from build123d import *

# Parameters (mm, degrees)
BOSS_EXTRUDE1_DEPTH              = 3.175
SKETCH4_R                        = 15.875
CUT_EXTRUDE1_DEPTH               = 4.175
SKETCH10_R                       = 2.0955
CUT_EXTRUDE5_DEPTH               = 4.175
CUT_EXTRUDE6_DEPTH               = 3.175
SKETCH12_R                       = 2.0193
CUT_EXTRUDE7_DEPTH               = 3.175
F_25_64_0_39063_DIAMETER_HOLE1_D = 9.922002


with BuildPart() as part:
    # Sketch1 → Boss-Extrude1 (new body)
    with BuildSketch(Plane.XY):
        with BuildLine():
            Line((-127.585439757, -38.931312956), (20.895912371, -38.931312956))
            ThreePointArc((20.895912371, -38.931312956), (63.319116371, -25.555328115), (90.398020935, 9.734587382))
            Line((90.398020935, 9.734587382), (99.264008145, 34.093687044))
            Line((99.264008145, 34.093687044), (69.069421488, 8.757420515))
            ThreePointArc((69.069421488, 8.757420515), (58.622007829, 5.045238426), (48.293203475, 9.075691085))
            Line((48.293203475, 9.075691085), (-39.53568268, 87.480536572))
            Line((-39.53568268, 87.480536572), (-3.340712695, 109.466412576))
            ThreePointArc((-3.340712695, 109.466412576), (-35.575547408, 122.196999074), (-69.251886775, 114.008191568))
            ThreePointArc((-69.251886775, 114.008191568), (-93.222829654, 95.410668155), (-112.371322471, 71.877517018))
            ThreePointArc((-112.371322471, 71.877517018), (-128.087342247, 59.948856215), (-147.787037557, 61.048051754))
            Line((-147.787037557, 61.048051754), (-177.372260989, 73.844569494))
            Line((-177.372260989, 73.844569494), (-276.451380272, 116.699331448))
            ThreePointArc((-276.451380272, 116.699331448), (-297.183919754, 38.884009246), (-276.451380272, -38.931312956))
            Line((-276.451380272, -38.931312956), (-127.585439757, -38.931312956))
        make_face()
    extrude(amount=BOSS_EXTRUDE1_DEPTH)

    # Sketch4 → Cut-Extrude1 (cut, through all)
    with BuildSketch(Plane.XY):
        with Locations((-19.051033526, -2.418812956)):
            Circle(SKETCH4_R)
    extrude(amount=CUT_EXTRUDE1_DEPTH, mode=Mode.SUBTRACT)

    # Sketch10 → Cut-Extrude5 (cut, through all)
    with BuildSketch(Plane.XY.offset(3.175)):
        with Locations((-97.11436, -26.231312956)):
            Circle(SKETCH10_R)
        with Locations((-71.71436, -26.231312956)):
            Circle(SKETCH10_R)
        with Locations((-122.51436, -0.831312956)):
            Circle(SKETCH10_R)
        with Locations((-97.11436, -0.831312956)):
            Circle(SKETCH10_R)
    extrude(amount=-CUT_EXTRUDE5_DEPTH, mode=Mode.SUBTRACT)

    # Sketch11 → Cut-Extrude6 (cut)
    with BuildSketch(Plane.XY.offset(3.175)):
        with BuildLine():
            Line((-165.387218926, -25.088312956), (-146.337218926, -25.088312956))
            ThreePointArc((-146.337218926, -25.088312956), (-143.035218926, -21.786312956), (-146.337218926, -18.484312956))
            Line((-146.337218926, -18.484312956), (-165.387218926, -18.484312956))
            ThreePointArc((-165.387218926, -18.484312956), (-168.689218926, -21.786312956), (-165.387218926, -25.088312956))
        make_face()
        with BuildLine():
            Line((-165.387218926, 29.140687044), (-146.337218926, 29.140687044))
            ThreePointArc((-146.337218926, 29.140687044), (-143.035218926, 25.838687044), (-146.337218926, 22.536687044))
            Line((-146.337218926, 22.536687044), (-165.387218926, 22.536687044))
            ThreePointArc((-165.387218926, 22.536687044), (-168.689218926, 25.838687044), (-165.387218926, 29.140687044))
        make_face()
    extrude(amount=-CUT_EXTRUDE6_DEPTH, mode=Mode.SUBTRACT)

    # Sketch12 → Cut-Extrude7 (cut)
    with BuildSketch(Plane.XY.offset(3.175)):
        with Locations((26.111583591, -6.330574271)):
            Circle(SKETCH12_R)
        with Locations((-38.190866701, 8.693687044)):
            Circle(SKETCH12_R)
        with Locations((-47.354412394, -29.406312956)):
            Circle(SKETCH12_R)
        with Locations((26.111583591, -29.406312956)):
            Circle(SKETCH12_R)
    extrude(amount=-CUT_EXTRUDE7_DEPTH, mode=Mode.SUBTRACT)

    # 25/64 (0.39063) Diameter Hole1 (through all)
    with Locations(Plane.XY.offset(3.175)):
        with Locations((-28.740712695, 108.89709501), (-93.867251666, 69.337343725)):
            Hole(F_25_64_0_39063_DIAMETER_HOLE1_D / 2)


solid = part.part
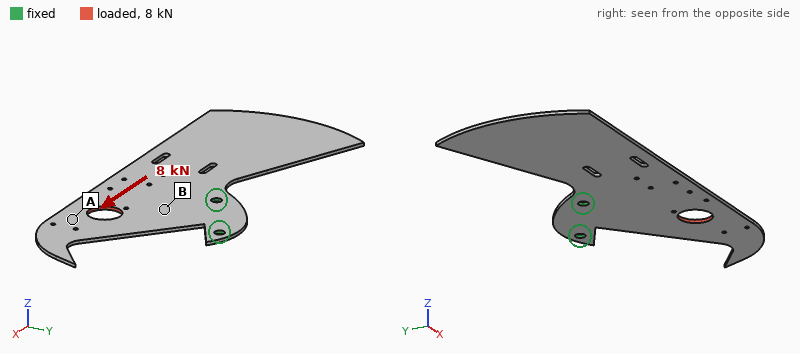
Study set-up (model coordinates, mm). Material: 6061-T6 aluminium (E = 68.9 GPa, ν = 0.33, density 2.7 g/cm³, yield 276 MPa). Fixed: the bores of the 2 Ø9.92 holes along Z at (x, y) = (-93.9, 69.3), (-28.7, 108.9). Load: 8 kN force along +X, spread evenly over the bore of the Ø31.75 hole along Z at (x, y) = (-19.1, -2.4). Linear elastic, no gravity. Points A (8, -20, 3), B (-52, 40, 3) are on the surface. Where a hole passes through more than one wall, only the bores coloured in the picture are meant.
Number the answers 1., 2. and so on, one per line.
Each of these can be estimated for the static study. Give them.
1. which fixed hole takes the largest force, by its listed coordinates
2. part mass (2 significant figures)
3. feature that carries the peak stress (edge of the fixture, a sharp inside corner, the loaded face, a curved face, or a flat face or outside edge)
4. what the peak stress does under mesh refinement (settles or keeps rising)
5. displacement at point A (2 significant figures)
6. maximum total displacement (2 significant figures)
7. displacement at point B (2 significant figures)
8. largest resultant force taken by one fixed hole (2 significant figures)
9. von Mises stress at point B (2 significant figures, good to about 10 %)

1. (-93.9, 69.3)
2. 350 g
3. edge of the fixture
4. keeps rising
5. 0.62 mm
6. 1.0 mm
7. 0.20 mm
8. 12 kN
9. 78 MPa
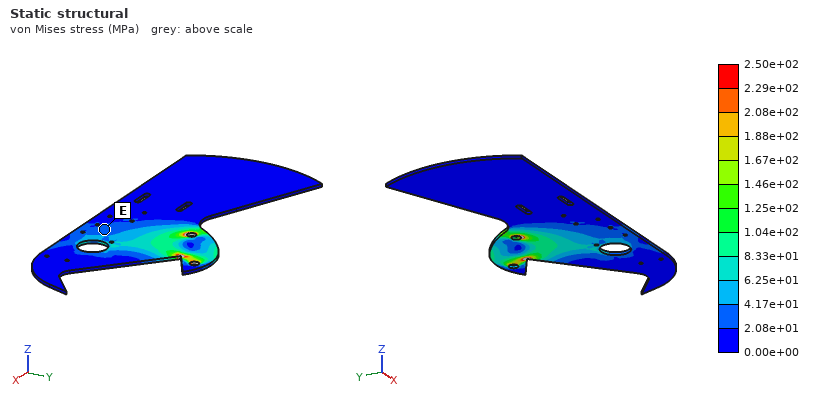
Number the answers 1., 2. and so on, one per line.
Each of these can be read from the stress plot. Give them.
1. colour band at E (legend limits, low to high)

1. 2.08e+01 to 4.17e+01 MPa
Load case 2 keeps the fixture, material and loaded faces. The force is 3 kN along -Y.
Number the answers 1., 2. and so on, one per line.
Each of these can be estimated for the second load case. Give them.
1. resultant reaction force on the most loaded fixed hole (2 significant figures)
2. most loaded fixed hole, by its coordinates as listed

1. 2.9 kN
2. (-28.7, 108.9)
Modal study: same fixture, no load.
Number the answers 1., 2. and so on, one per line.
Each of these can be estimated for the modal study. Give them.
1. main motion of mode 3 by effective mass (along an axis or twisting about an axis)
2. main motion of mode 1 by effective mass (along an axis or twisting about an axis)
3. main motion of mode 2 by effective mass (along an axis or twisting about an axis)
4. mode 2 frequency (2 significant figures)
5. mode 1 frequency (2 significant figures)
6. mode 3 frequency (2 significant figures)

1. twisting about X
2. along Z
3. along Z
4. 100 Hz
5. 46 Hz
6. 130 Hz
